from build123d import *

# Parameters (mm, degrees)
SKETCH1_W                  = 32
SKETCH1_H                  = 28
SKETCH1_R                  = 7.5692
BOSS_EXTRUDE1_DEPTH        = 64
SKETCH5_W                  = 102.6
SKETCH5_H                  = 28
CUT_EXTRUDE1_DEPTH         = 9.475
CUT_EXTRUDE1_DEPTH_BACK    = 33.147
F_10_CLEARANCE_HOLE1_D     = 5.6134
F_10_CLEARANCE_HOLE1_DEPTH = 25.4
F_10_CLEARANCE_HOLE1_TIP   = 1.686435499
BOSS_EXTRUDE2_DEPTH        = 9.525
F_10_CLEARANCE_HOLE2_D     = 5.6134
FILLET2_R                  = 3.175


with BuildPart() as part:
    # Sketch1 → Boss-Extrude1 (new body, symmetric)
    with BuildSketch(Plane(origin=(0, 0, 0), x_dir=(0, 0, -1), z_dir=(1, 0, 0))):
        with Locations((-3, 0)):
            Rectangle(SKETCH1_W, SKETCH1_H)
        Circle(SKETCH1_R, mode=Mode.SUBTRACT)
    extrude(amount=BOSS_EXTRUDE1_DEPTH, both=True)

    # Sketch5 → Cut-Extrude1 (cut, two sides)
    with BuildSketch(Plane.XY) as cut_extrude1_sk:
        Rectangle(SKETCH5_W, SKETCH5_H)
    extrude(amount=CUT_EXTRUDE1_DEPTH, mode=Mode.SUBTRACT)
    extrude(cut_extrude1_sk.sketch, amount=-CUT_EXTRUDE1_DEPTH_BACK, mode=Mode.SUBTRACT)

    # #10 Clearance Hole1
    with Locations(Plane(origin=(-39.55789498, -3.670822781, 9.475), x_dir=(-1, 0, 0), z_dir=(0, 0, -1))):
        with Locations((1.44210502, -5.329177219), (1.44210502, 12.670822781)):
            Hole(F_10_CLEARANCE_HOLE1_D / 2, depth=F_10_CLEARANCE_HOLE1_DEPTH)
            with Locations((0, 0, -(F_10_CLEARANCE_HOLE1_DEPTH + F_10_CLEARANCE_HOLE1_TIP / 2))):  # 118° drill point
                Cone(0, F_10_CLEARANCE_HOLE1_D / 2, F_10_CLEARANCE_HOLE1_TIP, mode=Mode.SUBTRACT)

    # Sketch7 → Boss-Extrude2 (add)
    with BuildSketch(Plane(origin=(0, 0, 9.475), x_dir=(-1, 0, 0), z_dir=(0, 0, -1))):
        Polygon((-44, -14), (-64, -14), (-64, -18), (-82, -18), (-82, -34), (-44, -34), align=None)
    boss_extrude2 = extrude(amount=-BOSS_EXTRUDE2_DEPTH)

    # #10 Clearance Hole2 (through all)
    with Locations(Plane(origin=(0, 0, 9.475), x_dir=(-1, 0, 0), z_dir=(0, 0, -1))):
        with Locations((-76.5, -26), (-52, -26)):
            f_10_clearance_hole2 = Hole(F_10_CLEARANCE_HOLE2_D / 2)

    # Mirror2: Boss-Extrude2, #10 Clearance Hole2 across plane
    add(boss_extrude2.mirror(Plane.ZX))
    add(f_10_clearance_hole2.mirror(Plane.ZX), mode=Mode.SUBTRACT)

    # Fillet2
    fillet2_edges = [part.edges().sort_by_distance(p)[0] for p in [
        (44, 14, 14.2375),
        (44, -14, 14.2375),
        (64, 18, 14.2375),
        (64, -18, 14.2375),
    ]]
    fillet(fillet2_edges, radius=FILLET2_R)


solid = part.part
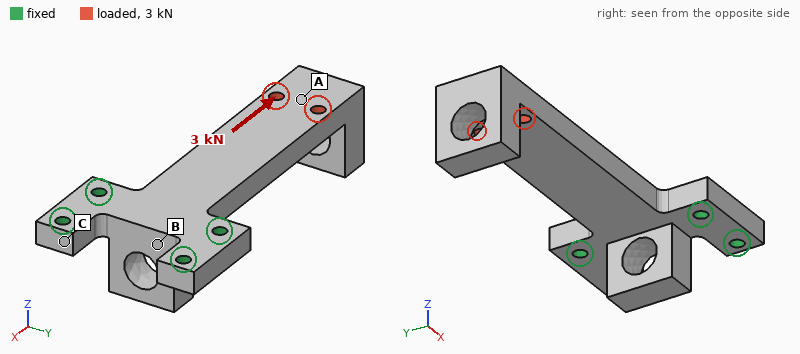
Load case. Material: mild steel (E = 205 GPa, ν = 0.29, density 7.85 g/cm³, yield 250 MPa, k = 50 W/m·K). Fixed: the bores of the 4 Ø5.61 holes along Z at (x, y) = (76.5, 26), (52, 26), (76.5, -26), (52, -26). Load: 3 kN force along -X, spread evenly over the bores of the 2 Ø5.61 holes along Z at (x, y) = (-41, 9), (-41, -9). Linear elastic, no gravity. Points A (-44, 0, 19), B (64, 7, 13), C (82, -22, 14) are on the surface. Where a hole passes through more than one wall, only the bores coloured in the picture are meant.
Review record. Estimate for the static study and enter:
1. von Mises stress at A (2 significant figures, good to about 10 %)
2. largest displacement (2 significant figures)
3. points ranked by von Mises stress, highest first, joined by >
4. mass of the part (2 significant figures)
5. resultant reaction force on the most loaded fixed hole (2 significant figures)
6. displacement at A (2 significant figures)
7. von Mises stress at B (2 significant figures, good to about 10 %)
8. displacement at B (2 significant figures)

5.5 MPa
7.1 µm
B > A > C
450 g
1.1 kN
6.7 µm
9.2 MPa
1.8 µm
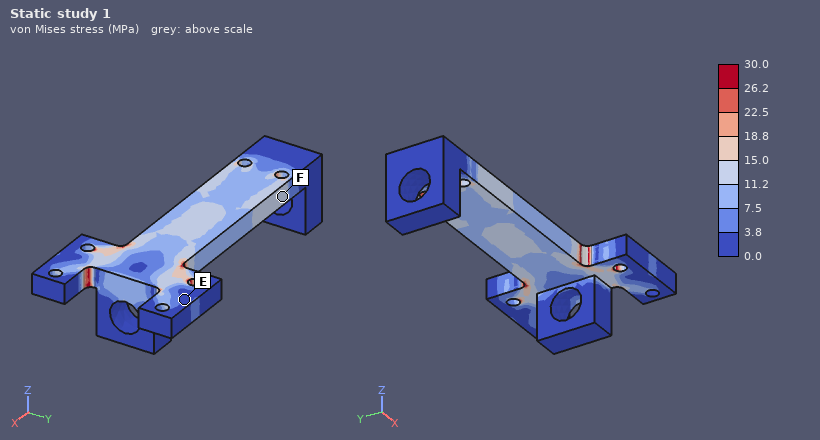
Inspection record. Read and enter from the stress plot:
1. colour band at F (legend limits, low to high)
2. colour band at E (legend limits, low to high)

11.2 to 15.0 MPa
0.0 to 3.8 MPa
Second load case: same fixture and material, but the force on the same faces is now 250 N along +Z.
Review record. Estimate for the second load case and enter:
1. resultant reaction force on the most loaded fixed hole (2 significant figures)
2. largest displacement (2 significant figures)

400 N
0.27 mm
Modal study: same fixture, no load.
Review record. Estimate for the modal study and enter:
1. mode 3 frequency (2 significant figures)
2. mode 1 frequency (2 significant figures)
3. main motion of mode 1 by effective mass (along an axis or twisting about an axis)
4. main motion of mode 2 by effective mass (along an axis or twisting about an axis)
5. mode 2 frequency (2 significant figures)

2500 Hz
420 Hz
along Z
along Y
1200 Hz
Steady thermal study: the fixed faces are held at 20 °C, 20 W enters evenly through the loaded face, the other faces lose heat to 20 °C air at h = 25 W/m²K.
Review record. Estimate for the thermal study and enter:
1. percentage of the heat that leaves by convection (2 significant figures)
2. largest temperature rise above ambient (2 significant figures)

63 %
73 K
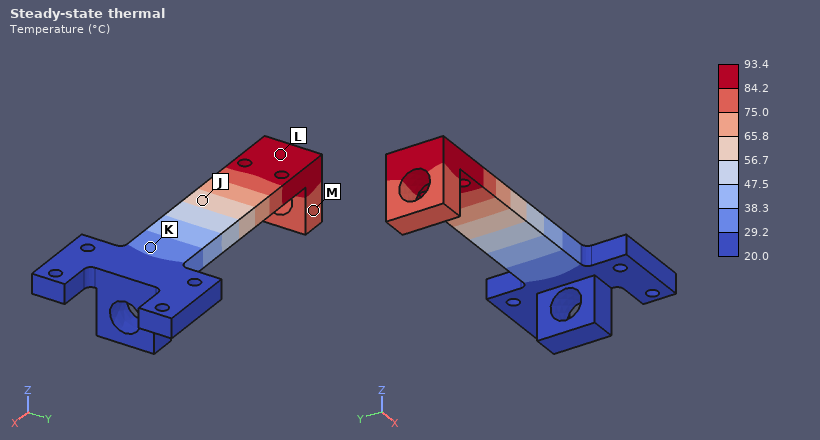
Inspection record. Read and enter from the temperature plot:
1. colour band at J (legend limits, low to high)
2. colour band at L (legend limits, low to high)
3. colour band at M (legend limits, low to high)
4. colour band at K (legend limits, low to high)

56.7 to 65.8 °C
84.2 to 93.4 °C
75.0 to 84.2 °C
29.2 to 38.3 °C
